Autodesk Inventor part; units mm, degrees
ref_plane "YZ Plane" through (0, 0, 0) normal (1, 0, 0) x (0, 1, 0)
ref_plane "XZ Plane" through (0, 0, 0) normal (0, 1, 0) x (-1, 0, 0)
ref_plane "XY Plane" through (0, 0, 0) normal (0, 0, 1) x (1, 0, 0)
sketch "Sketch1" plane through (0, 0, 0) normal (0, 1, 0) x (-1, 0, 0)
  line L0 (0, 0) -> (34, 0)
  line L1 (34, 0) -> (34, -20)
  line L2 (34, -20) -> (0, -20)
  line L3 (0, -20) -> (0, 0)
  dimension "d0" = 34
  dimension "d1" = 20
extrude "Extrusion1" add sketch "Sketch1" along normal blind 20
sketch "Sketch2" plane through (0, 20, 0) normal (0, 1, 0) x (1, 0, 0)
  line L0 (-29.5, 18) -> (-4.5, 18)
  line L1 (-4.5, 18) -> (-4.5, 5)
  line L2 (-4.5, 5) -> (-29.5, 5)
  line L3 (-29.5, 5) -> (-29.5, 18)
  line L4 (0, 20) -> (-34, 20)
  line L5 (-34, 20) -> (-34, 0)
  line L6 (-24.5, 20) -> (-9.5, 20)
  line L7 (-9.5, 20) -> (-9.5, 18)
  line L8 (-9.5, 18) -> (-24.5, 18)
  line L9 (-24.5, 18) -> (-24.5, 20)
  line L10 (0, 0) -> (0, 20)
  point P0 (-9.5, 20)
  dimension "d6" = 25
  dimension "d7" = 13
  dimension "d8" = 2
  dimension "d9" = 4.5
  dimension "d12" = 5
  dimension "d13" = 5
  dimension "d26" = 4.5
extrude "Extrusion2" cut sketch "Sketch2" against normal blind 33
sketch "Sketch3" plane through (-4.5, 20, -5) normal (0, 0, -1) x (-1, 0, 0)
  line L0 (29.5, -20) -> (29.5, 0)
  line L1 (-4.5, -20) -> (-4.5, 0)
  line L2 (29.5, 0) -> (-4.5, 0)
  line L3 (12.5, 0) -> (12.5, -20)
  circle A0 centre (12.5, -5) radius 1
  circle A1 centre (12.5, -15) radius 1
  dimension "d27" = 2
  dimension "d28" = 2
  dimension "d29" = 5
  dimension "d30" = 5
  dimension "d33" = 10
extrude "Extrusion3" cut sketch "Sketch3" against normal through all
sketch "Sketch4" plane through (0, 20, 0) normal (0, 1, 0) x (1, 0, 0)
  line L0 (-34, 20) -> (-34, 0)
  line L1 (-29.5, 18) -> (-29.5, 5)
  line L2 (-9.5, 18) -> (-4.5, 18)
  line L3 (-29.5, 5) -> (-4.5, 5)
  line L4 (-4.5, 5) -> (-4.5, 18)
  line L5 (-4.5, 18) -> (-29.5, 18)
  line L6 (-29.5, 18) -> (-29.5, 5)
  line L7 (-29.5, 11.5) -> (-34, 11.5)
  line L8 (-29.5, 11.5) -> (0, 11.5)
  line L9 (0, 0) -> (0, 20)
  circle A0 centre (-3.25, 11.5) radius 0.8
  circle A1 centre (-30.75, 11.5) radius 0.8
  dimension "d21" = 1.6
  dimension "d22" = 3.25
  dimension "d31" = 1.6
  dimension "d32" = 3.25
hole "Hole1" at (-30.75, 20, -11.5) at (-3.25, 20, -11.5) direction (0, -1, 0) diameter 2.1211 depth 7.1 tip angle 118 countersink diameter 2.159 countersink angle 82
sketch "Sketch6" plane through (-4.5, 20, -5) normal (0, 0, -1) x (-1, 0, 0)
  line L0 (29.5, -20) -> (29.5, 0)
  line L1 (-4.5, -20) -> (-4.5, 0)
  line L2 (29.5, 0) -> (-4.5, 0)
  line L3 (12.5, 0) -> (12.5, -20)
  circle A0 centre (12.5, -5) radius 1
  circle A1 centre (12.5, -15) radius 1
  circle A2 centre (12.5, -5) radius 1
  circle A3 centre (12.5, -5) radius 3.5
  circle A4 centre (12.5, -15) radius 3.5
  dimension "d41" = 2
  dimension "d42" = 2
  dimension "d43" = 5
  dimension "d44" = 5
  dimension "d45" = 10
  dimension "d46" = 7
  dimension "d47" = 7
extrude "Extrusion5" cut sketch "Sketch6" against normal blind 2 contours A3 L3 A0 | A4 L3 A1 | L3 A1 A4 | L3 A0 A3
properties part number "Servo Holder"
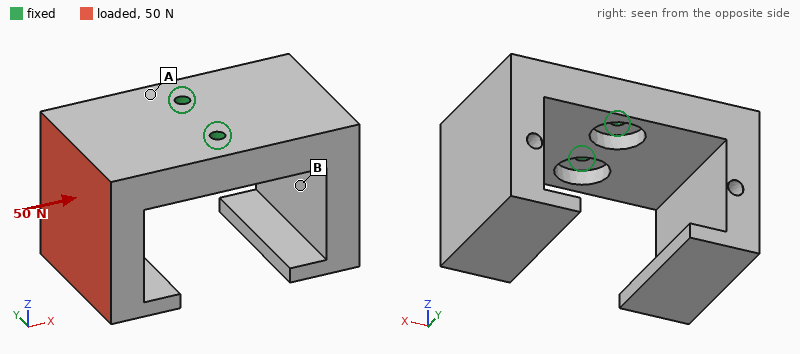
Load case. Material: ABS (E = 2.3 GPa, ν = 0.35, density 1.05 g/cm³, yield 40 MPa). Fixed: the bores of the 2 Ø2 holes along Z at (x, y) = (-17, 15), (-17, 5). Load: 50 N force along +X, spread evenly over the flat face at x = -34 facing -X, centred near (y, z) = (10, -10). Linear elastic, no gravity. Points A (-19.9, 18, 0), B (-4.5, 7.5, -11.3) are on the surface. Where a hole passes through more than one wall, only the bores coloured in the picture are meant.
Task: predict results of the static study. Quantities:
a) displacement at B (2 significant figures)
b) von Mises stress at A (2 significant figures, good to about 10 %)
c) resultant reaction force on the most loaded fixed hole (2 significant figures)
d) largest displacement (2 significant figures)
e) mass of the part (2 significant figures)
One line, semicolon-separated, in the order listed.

0.084 mm; 5.6 MPa; 25 N; 0.47 mm; 6.6 g
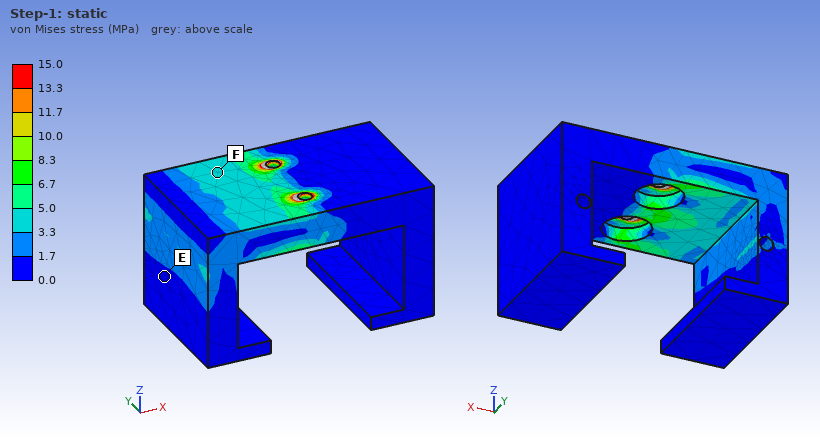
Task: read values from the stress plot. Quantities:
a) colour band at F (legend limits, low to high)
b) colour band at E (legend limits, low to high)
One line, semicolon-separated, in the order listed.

3.3 to 5.0 MPa; 0.0 to 1.7 MPa
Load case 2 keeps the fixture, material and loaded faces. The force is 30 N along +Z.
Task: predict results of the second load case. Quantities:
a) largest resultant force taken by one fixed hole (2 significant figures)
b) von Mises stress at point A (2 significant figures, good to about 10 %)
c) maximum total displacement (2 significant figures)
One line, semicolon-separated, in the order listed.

15 N; 6.3 MPa; 0.41 mm
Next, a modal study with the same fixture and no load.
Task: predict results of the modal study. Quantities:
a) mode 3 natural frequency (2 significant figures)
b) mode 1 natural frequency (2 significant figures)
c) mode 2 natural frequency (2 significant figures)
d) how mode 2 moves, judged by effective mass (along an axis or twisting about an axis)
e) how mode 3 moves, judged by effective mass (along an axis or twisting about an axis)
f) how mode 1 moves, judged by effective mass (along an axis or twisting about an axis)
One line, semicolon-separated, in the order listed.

1900 Hz; 880 Hz; 1300 Hz; along Z; twisting about Z; along X
